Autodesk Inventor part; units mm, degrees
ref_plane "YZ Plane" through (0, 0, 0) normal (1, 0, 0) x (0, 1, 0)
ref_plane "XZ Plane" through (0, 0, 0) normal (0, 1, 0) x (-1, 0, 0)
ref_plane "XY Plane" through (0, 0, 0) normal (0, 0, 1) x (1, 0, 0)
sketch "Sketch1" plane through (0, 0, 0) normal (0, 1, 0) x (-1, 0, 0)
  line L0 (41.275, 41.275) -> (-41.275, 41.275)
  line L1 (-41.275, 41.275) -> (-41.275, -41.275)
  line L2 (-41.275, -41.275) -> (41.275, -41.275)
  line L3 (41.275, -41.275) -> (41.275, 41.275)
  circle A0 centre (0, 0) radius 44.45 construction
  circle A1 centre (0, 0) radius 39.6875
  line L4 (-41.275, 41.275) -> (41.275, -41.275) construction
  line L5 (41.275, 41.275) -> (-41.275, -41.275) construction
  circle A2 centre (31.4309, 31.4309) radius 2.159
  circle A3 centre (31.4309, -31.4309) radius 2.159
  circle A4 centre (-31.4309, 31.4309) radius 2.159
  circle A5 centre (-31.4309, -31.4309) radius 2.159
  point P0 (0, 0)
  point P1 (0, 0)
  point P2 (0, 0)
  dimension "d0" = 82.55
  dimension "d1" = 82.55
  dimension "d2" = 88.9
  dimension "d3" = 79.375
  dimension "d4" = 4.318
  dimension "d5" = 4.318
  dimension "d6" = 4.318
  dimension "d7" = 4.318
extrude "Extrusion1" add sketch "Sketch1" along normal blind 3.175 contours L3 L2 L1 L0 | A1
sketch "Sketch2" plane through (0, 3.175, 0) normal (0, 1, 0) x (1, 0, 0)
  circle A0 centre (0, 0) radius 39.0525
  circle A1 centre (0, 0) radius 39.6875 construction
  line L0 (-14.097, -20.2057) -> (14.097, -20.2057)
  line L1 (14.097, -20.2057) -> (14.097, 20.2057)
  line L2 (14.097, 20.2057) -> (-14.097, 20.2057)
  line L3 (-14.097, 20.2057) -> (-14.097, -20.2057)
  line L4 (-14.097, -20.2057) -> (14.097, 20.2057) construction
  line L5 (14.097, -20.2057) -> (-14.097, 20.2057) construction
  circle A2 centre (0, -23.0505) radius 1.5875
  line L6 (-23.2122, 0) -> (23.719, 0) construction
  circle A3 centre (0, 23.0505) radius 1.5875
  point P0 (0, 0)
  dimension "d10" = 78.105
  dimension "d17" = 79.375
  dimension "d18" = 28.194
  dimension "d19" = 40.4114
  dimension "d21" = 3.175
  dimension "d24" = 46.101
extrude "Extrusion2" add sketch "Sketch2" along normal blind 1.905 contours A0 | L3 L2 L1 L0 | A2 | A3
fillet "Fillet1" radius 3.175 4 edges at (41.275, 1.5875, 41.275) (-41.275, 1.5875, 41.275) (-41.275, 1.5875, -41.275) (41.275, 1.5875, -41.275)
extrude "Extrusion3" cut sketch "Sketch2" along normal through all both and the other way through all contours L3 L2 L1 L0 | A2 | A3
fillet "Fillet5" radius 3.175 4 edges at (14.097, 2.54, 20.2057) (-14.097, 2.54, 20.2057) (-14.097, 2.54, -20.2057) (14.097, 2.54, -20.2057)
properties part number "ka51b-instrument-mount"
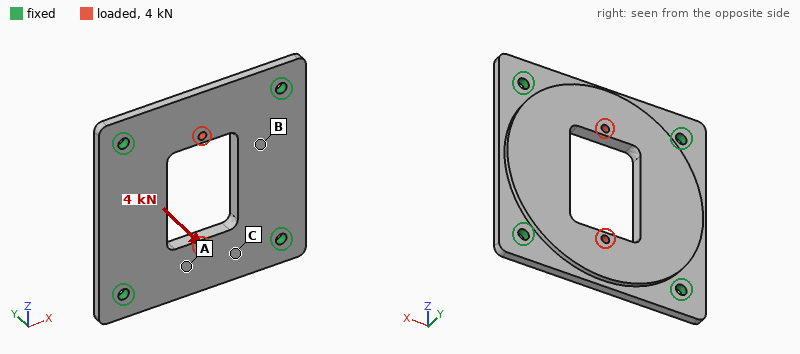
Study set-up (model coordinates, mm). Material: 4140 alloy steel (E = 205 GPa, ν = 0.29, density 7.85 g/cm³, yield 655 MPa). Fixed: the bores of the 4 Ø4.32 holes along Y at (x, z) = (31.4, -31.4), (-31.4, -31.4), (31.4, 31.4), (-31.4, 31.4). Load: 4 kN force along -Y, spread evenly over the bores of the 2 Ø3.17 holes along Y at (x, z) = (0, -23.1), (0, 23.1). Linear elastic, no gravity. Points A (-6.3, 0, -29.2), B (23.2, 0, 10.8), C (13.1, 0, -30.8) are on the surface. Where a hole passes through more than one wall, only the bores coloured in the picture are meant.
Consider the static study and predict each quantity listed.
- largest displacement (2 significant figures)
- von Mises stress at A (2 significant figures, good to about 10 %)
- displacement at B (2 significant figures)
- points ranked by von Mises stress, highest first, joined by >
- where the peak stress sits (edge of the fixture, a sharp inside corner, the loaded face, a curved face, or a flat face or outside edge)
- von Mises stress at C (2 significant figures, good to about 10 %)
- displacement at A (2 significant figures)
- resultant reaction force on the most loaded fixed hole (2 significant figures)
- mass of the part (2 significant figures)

0.14 mm
150 MPa
0.055 mm
A > C > B
the loaded face
80 MPa
0.090 mm
2.2 kN
190 g
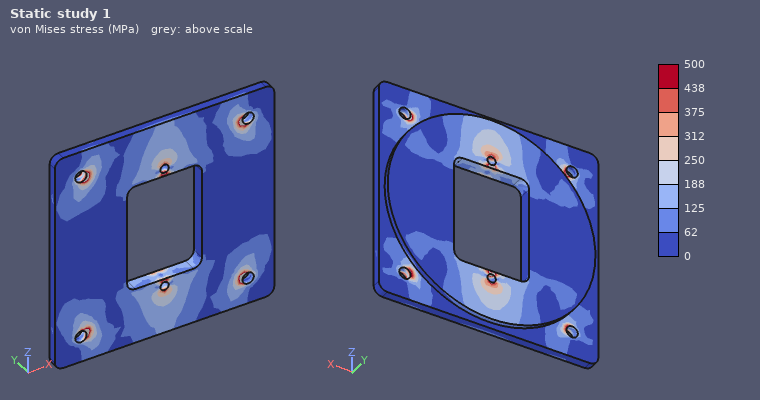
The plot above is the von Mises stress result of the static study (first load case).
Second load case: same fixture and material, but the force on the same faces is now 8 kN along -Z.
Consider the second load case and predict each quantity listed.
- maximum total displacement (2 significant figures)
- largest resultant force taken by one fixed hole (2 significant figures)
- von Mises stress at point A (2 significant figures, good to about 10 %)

17 µm
2.1 kN
53 MPa
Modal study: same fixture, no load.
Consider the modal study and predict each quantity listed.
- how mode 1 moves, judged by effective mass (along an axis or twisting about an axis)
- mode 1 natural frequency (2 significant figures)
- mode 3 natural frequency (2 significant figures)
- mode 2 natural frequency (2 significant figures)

along Y
4000 Hz
5300 Hz
5300 Hz
